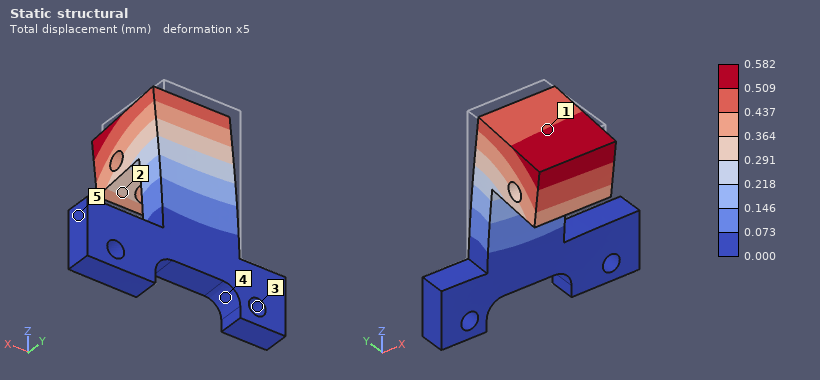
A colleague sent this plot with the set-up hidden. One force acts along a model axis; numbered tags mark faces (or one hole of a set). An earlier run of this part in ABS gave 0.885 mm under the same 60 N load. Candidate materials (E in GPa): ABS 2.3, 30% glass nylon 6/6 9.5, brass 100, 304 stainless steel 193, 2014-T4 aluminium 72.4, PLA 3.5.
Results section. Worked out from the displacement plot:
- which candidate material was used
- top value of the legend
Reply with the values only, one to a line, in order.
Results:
PLA
0.582 mm
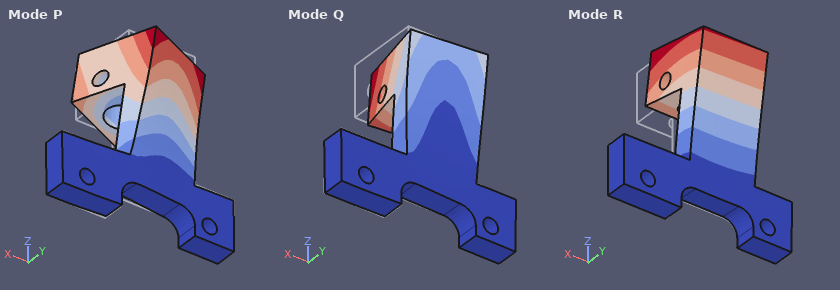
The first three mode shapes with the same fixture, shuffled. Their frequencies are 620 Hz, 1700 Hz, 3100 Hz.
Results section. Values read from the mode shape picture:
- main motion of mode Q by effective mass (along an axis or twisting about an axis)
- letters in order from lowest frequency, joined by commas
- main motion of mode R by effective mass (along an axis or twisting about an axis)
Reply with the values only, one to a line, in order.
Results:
along X
R, Q, P
along Y
